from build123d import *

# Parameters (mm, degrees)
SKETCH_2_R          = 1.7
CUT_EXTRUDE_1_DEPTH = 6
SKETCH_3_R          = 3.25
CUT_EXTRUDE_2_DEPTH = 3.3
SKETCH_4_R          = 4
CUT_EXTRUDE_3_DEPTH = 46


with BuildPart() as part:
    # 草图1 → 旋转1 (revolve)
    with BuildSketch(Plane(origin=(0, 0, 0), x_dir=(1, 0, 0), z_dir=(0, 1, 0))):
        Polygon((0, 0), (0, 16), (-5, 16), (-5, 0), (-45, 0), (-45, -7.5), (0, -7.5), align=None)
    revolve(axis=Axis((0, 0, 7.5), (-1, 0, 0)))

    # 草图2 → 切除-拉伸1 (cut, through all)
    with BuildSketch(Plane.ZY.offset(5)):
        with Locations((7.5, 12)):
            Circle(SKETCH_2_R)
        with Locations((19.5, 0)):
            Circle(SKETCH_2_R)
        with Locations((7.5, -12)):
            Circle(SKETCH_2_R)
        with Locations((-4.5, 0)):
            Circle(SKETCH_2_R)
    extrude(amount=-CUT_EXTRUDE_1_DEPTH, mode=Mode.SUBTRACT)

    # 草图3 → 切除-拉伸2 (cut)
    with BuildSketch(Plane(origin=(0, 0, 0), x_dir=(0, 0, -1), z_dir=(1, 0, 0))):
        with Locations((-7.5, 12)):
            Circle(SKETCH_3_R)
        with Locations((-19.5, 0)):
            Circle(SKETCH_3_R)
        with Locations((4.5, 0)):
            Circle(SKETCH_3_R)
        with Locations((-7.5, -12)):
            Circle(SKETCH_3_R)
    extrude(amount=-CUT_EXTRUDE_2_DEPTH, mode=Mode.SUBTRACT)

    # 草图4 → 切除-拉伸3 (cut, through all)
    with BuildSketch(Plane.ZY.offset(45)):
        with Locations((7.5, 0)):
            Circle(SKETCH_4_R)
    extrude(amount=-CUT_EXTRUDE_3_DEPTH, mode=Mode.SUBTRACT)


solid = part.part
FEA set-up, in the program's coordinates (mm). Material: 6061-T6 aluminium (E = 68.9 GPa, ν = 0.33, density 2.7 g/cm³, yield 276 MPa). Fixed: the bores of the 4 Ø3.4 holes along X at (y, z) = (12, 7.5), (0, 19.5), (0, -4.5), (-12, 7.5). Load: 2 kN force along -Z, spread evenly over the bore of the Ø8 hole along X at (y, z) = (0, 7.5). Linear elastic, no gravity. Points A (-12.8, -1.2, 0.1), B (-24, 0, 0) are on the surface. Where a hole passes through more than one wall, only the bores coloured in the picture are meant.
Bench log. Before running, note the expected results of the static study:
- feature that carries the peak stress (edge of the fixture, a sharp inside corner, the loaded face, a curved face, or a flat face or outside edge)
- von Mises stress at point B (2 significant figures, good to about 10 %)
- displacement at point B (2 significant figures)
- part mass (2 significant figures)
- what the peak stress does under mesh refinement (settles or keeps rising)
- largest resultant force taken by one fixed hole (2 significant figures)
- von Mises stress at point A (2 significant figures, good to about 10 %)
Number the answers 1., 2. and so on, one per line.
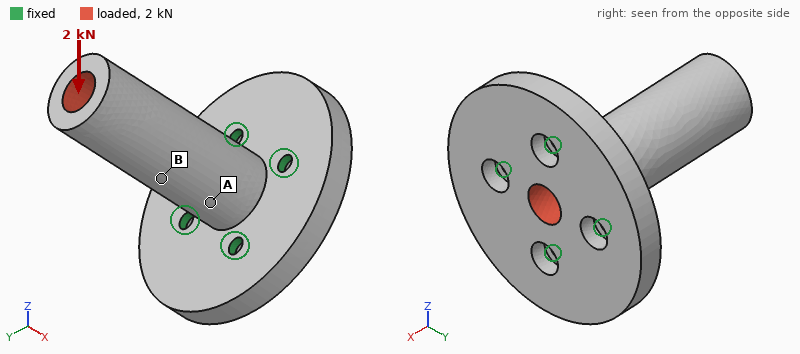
1. edge of the fixture
2. 32 MPa
3. 0.10 mm
4. 35 g
5. keeps rising
6. 1.6 kN
7. 70 MPa
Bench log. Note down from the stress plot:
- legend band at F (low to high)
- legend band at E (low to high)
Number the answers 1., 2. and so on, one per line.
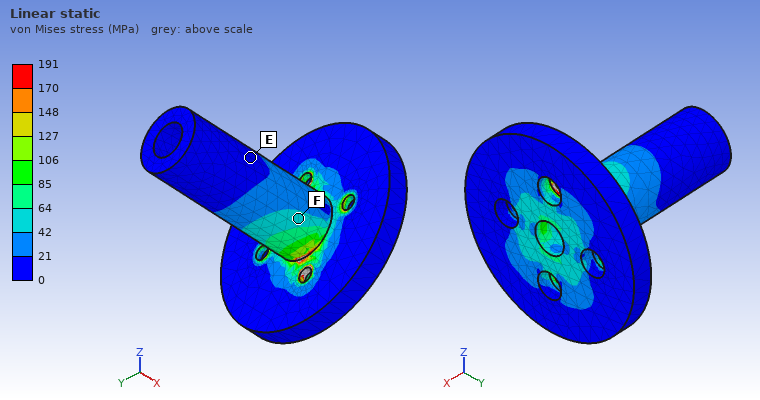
1. 42 to 64 MPa
2. 0 to 21 MPa
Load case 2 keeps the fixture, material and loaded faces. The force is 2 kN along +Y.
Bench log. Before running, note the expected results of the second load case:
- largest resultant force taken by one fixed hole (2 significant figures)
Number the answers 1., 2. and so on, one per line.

1. 1.6 kN
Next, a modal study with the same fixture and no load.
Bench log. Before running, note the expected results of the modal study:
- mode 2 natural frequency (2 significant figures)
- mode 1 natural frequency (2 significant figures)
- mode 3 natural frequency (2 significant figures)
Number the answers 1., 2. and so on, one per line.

1. 4800 Hz
2. 4800 Hz
3. 13 kHz
